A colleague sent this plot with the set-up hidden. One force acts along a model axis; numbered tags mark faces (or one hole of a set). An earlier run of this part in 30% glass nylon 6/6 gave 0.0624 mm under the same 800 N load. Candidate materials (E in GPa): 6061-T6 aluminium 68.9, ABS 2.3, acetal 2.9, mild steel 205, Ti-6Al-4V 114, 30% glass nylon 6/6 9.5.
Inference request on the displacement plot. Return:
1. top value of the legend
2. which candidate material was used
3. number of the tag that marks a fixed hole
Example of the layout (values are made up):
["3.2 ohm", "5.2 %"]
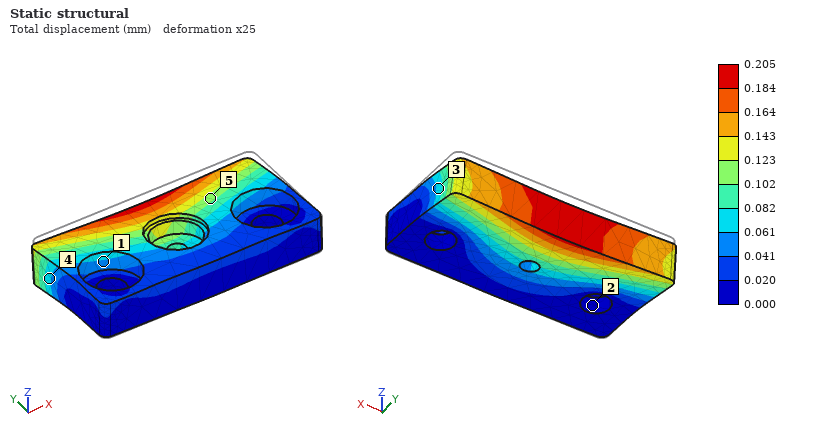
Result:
["0.205 mm", "acetal", "2"]
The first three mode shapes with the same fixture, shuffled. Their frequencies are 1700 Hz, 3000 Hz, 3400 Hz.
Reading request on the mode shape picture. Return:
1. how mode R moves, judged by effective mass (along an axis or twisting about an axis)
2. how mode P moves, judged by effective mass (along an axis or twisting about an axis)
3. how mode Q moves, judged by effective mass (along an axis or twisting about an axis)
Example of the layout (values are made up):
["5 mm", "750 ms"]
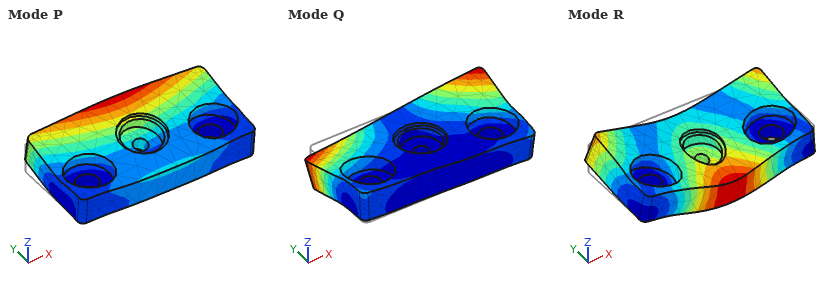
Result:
["along Z", "along Z", "twisting about Y"]
